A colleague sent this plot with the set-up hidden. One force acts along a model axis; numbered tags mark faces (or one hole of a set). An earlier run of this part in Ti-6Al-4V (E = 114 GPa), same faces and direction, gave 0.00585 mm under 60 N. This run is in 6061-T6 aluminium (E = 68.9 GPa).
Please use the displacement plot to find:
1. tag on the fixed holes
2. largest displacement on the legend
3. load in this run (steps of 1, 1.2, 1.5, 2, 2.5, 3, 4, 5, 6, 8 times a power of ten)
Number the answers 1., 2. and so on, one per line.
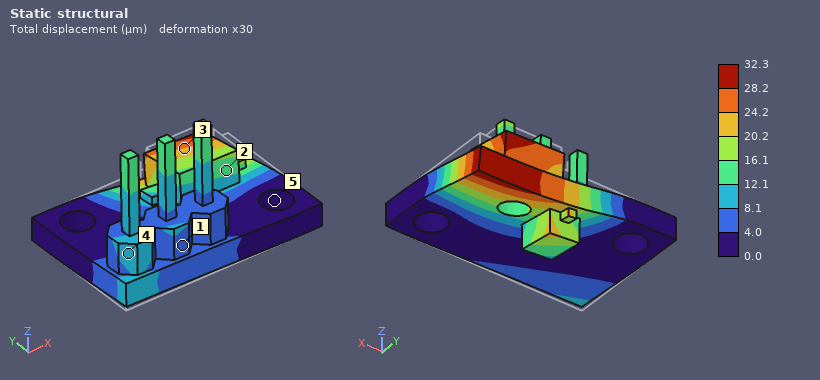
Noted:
1. 5
2. 32.3 µm
3. 200 N
